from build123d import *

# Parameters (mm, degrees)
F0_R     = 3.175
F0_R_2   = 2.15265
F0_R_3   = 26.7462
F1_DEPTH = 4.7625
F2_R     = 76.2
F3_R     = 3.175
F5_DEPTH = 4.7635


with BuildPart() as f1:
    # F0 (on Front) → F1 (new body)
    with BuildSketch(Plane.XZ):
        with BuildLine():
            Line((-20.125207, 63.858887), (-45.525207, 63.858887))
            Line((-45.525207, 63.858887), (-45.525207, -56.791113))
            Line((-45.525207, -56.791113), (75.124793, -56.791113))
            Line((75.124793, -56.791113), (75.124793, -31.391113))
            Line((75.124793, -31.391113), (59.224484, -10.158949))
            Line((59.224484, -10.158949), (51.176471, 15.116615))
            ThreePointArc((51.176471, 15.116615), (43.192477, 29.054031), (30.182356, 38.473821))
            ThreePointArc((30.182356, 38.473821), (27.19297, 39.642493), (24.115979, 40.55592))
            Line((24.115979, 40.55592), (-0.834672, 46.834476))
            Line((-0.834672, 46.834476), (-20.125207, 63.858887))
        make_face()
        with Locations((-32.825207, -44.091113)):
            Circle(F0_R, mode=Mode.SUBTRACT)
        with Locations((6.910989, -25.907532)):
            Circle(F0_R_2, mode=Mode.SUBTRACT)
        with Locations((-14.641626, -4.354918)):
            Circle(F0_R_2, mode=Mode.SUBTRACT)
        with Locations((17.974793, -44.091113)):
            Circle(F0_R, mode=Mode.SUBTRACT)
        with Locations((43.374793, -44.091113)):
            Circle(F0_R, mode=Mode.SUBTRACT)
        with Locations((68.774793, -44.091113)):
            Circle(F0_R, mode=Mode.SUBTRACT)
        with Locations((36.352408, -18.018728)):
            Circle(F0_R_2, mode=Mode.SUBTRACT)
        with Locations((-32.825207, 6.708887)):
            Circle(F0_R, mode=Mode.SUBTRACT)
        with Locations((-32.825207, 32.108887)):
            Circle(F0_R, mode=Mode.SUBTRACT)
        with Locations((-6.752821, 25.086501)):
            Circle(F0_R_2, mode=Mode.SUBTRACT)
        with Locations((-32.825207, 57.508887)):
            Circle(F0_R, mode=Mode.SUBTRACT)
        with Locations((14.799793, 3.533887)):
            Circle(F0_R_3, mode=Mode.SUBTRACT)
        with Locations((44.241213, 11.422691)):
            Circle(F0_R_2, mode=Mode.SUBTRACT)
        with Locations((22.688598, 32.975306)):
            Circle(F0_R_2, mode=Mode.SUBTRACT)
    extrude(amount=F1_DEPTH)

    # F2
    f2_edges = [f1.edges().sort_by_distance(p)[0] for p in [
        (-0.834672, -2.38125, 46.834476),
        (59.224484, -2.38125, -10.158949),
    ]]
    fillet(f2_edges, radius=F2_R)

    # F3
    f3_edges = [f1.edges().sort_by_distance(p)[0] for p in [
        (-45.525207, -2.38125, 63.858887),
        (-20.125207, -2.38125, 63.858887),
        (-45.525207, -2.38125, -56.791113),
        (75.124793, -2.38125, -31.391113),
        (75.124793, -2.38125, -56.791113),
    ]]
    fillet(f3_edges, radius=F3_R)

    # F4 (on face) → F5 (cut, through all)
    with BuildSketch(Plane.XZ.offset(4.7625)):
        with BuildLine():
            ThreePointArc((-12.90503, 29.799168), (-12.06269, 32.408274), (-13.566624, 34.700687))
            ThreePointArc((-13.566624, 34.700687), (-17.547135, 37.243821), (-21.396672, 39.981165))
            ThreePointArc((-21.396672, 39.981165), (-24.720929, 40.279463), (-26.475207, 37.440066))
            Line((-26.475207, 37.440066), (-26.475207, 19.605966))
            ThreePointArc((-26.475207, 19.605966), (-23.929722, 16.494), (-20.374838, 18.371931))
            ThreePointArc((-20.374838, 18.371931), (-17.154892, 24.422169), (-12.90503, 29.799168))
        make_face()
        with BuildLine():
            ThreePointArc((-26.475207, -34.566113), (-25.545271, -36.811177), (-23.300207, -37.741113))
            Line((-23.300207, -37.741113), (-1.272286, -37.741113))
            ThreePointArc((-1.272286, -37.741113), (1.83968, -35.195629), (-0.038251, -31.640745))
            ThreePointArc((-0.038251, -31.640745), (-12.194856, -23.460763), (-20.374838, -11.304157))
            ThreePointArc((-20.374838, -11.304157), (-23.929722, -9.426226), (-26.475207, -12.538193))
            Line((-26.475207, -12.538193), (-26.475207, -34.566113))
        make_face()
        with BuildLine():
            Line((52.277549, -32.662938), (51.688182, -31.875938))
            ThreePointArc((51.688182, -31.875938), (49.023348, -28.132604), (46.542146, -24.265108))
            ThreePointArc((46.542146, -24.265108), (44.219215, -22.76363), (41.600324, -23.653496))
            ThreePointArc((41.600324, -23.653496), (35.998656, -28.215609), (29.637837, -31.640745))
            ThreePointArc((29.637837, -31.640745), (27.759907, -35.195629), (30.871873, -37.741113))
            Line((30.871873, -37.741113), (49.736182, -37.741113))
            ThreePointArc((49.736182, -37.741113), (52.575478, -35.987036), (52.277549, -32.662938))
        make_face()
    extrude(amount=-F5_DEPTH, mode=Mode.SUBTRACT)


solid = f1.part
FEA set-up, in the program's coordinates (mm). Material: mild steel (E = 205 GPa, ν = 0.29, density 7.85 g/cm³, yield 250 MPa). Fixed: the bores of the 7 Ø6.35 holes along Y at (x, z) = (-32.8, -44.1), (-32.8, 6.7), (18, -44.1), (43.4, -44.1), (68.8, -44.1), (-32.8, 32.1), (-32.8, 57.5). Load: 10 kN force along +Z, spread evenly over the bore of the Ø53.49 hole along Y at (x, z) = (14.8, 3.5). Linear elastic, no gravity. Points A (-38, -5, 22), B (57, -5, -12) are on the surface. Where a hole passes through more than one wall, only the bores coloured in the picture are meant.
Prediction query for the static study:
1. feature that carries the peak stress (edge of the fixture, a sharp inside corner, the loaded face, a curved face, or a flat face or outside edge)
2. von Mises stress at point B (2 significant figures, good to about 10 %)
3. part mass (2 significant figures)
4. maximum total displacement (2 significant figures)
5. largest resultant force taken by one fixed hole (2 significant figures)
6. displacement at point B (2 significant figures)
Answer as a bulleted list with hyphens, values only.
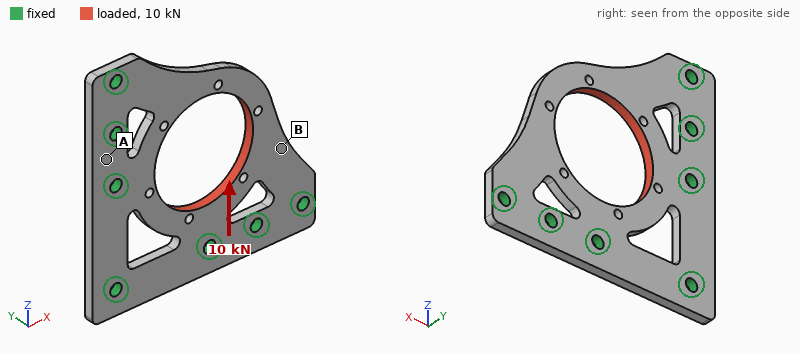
- a curved face
- 33 MPa
- 290 g
- 21 µm
- 3.1 kN
- 5.2 µm
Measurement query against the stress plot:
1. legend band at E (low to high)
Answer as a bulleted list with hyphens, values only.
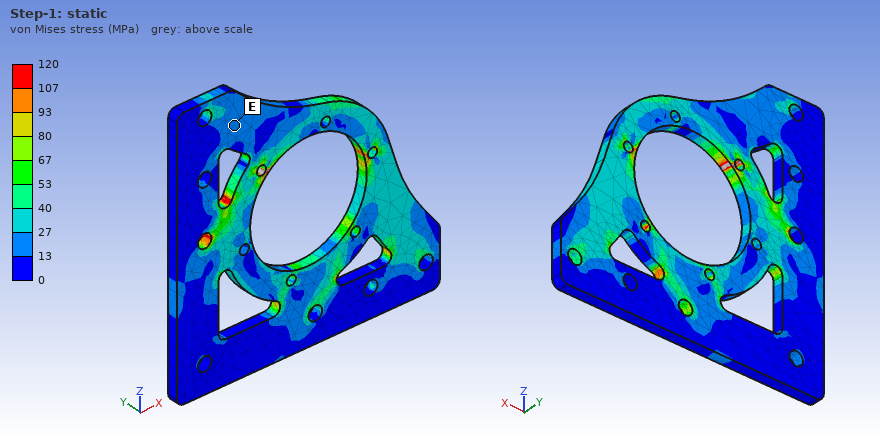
- 13 to 27 MPa
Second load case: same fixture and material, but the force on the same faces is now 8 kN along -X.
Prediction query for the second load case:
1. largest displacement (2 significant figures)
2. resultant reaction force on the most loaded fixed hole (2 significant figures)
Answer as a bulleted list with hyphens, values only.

- 17 µm
- 2.4 kN
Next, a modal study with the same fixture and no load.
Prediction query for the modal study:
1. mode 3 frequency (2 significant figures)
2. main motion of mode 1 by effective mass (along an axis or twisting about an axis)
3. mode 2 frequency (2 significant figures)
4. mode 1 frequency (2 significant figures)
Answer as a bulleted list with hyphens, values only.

- 5500 Hz
- along Y
- 3300 Hz
- 1400 Hz
